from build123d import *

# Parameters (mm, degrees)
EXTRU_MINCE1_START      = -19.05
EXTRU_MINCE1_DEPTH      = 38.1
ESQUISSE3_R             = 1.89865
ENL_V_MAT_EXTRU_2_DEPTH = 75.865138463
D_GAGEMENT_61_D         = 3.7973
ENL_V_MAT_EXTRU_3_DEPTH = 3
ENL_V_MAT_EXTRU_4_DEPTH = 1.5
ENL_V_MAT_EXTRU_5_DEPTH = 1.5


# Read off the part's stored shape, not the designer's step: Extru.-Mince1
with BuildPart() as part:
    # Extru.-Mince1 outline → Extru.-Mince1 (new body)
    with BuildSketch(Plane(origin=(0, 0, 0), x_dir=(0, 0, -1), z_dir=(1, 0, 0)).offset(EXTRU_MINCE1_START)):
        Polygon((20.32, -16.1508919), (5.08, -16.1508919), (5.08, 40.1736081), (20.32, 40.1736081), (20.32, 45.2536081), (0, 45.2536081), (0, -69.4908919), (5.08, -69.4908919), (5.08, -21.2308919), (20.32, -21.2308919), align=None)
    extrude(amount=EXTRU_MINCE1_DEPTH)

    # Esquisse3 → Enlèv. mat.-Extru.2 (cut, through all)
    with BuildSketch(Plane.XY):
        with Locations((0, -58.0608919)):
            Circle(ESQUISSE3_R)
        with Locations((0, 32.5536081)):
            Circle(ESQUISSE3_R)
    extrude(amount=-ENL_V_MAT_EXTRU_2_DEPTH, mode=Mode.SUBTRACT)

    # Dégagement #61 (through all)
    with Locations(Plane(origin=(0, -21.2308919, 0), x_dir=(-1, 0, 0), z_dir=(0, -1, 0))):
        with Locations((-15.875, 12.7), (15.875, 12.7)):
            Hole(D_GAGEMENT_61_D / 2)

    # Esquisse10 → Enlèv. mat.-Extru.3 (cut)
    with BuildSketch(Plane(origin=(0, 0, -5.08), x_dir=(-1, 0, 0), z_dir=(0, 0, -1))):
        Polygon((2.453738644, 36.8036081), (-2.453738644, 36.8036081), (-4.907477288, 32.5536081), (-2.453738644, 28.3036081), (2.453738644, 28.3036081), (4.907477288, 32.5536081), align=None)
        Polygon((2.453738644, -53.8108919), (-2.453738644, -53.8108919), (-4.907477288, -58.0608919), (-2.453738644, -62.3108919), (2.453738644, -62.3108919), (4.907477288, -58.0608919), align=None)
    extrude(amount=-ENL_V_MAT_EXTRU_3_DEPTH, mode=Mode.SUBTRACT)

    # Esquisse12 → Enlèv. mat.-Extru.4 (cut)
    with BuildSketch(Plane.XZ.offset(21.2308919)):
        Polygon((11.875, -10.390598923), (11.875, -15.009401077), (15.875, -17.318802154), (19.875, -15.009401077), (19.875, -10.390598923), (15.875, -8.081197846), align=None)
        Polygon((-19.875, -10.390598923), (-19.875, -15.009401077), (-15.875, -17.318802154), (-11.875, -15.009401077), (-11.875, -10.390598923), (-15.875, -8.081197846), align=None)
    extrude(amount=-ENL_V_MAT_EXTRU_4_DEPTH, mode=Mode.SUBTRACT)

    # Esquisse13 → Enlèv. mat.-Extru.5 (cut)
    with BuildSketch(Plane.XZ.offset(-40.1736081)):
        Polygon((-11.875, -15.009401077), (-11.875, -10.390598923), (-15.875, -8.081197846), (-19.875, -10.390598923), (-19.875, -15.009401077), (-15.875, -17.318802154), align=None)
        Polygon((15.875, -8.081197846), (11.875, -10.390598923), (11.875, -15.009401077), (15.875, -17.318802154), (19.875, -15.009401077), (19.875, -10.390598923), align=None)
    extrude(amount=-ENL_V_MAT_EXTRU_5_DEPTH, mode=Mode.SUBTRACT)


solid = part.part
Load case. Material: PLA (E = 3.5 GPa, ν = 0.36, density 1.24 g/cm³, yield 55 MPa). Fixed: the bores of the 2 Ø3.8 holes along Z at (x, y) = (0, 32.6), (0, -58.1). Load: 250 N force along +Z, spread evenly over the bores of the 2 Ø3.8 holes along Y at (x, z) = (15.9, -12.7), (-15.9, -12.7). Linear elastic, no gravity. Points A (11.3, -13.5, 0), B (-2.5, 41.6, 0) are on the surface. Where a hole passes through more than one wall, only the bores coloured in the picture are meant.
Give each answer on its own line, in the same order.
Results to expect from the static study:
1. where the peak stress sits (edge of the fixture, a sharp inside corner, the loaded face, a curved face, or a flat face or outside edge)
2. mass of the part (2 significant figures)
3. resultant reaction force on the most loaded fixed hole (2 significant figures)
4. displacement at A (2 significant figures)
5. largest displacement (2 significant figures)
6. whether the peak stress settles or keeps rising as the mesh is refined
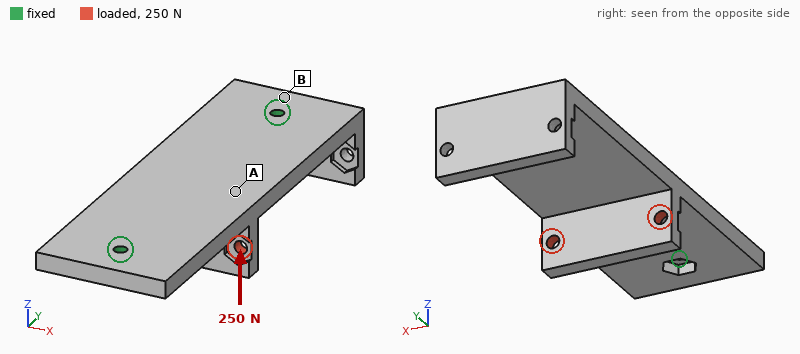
edge of the fixture
34 g
420 N
1.1 mm
1.2 mm
keeps rising
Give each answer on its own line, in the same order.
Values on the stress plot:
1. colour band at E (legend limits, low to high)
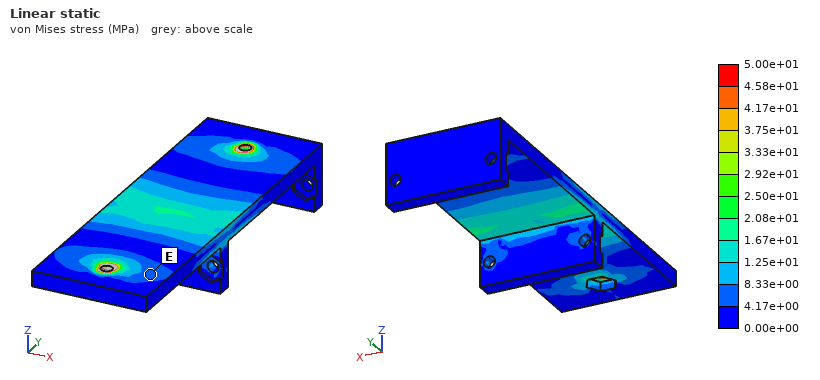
4.17e+00 to 8.33e+00 MPa
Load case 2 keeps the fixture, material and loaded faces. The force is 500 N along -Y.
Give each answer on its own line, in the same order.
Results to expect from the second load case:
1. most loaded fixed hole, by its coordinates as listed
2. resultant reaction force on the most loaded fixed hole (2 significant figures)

(0, 32.6)
290 N
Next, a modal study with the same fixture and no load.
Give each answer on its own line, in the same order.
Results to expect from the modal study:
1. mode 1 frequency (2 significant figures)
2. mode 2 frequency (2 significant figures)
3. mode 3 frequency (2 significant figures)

620 Hz
630 Hz
1200 Hz
